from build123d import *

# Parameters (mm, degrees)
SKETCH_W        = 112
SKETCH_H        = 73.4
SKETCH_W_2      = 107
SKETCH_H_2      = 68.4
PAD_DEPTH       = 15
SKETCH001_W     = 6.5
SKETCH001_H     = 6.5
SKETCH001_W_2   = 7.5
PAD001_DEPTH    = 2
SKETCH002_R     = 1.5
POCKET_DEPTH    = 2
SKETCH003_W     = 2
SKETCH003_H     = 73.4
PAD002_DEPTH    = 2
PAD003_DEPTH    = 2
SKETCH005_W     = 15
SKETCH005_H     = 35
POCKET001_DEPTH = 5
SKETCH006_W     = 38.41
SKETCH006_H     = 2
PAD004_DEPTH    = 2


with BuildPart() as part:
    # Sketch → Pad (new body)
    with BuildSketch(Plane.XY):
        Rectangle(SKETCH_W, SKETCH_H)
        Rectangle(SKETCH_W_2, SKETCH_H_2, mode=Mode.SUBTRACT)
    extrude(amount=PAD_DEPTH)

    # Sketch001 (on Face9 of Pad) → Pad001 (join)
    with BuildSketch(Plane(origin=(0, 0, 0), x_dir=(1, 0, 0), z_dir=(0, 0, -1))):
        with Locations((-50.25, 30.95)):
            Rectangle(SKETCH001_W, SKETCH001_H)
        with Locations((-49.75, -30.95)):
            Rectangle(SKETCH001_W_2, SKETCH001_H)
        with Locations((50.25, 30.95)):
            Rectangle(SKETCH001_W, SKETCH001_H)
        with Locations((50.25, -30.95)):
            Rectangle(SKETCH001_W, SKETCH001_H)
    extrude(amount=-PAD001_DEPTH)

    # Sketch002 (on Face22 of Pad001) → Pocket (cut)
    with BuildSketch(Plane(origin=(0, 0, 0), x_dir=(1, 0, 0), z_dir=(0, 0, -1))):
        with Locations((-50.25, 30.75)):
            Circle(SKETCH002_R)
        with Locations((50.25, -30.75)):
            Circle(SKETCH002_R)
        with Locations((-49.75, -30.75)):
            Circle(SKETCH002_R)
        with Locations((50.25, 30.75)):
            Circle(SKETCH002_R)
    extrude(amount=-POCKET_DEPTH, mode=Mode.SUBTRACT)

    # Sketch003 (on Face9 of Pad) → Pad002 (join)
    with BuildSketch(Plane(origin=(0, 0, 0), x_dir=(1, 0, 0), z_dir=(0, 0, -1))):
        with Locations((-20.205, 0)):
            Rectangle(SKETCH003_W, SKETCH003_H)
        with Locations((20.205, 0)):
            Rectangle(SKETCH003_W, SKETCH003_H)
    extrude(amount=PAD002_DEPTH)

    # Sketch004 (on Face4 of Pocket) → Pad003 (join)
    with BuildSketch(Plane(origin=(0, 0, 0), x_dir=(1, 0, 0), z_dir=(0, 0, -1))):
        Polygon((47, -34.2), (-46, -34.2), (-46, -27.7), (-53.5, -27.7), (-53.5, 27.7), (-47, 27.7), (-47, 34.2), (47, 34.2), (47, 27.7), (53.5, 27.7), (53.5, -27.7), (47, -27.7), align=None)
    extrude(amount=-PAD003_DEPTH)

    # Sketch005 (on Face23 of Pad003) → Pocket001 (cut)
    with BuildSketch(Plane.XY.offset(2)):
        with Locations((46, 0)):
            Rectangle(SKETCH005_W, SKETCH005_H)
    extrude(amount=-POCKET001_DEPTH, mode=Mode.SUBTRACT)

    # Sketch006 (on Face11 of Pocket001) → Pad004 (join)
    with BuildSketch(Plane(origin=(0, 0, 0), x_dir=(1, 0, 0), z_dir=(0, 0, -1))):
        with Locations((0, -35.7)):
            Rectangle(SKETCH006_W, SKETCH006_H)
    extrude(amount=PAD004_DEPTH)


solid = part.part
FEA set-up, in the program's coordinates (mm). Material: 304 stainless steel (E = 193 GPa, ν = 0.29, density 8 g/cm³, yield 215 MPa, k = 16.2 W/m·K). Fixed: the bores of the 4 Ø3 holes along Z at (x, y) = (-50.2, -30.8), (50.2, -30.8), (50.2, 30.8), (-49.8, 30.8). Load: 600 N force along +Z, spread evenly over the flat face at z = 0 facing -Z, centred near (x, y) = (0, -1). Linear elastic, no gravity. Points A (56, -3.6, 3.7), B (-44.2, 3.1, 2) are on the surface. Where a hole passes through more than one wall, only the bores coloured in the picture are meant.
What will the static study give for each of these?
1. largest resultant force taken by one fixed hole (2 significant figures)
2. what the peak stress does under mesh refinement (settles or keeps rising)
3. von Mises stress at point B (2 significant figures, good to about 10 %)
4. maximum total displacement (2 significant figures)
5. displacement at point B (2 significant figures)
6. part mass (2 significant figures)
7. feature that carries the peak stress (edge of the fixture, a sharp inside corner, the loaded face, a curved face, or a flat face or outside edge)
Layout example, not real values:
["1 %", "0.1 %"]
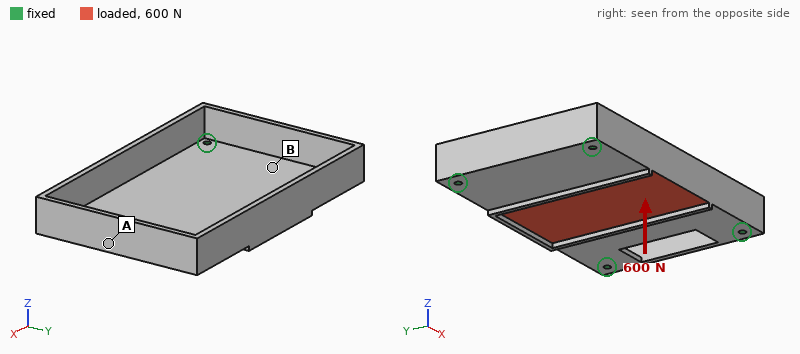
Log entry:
["280 N", "keeps rising", "16 MPa", "0.11 mm", "0.017 mm", "220 g", "edge of the fixture"]
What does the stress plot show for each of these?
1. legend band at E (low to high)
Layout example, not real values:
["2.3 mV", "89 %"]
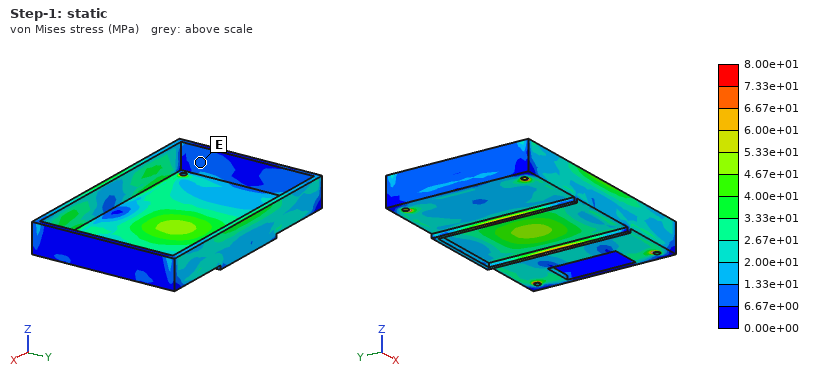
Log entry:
["6.67e+00 to 1.33e+01 MPa"]
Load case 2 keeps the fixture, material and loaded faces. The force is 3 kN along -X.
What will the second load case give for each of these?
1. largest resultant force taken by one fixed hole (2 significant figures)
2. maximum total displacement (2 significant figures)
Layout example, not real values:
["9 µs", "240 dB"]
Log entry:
["810 N", "10 µm"]
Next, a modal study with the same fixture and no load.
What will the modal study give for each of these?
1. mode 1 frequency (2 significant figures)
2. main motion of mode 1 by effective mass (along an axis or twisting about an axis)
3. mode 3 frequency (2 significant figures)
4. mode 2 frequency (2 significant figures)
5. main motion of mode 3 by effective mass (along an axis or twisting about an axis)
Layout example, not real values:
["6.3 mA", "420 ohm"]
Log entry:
["1600 Hz", "along Z", "3600 Hz", "2900 Hz", "twisting about X"]
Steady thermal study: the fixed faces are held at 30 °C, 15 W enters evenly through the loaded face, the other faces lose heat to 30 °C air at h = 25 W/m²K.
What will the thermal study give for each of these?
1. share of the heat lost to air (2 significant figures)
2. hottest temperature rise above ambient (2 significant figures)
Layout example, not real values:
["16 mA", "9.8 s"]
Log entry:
["80 %", "61 K"]
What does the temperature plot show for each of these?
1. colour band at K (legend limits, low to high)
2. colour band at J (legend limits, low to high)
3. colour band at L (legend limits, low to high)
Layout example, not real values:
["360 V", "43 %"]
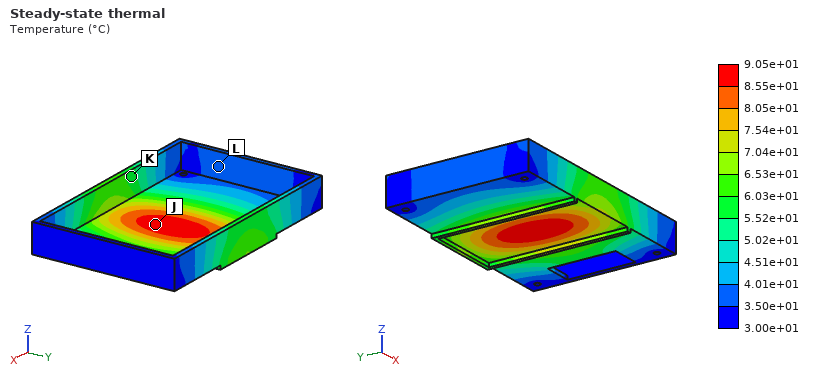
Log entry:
["5.52e+01 to 6.03e+01 °C", "8.55e+01 to 9.05e+01 °C", "3.50e+01 to 4.01e+01 °C"]
